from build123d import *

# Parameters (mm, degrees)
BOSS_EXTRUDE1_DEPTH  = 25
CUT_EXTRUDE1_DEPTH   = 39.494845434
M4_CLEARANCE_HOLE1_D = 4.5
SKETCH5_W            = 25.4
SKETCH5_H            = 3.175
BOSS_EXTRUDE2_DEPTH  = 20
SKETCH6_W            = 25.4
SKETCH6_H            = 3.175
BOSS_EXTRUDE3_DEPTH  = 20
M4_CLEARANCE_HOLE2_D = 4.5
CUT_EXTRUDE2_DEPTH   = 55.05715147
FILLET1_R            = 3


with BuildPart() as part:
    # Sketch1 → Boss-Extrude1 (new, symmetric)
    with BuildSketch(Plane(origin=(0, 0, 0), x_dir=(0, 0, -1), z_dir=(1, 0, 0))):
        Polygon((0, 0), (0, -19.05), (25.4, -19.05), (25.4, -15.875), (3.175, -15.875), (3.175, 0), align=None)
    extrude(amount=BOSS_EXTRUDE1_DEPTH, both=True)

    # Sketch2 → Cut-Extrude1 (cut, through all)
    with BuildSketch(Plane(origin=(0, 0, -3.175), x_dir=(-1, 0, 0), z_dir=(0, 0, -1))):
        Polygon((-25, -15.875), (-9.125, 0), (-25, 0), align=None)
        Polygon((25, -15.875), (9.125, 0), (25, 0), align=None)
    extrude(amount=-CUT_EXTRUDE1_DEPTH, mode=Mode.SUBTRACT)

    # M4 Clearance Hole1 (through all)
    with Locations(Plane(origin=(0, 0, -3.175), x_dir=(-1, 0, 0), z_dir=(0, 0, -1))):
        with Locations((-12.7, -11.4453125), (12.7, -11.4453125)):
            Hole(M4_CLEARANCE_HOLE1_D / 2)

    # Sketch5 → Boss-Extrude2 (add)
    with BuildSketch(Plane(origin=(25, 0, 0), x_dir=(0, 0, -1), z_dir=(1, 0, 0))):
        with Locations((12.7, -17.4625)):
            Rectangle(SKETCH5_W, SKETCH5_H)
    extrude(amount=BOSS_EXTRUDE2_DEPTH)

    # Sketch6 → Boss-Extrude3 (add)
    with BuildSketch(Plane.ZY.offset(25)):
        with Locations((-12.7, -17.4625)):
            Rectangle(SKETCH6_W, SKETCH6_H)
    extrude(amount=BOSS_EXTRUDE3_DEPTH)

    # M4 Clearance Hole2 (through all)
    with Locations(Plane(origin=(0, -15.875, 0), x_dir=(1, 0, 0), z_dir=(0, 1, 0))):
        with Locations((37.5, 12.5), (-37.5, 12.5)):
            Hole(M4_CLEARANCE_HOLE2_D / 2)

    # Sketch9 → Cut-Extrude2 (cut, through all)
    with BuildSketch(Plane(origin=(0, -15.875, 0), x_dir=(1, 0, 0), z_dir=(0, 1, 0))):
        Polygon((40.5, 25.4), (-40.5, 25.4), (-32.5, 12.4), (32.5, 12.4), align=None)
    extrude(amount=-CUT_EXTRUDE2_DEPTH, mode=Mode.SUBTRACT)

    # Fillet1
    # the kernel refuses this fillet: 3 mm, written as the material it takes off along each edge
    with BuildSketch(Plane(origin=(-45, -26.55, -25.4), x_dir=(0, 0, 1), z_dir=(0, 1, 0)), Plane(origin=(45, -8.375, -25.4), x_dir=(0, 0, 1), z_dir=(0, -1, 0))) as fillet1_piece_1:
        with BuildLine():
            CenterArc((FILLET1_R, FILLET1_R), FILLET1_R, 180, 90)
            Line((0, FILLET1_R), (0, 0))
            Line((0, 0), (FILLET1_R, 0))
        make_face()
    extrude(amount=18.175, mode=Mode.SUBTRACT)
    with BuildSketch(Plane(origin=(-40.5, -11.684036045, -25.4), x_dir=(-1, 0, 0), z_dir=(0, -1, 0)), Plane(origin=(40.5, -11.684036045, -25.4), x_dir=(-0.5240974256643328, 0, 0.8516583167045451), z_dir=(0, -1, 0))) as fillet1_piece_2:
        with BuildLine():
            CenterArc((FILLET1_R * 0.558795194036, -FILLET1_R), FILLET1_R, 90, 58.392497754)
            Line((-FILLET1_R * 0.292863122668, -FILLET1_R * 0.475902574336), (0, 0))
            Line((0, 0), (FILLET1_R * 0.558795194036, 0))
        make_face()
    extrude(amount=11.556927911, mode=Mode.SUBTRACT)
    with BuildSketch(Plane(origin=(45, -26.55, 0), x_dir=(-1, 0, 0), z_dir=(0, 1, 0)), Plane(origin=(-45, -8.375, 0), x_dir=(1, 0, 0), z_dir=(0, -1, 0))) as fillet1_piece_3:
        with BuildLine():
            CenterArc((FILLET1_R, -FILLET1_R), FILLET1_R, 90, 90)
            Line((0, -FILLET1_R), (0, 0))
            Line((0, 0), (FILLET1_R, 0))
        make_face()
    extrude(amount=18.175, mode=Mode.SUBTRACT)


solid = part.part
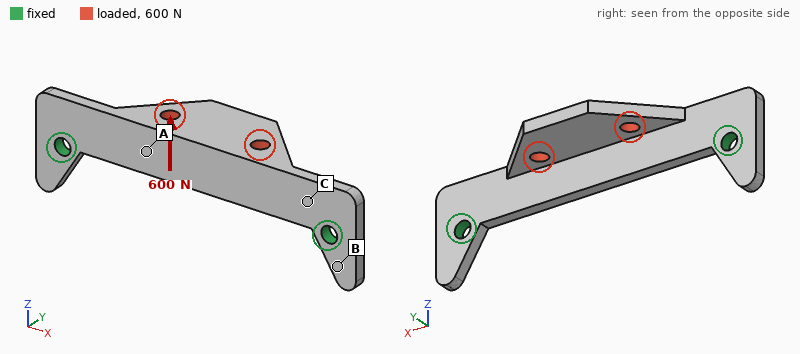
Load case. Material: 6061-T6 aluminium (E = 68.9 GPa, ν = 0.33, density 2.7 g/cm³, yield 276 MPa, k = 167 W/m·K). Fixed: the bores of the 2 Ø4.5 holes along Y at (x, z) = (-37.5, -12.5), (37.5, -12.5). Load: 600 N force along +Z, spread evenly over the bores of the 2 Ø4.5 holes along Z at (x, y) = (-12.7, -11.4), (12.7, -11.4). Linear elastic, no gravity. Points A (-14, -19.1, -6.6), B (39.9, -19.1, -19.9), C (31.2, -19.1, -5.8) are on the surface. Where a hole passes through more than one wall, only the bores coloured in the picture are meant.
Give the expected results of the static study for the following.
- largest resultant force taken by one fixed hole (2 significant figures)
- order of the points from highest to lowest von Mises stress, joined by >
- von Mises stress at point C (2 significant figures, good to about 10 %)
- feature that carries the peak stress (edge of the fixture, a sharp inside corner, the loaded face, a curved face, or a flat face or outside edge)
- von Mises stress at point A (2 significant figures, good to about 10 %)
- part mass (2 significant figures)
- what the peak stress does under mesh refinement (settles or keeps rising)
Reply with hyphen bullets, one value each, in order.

- 460 N
- C > A > B
- 60 MPa
- edge of the fixture
- 27 MPa
- 15 g
- keeps rising
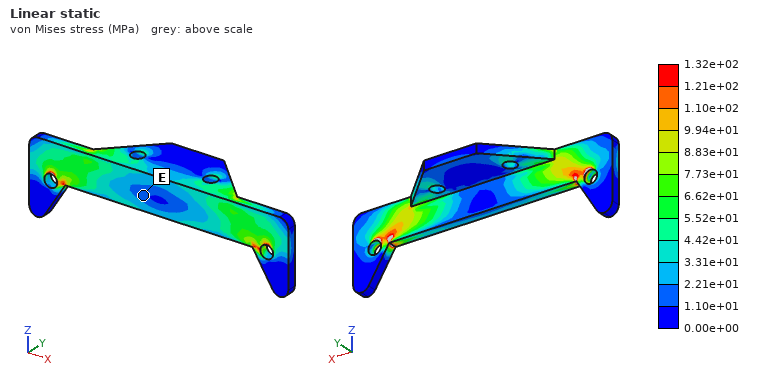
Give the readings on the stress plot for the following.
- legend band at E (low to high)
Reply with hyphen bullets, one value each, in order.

- 1.10e+01 to 2.21e+01 MPa
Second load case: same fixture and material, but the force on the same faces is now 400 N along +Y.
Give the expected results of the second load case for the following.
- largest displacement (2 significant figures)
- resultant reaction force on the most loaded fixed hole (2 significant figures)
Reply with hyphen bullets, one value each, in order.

- 0.16 mm
- 210 N
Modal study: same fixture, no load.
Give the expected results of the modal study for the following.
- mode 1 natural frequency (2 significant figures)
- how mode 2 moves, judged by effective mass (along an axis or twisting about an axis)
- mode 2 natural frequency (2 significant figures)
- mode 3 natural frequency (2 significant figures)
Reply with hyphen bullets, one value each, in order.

- 3000 Hz
- along Y
- 4200 Hz
- 7900 Hz
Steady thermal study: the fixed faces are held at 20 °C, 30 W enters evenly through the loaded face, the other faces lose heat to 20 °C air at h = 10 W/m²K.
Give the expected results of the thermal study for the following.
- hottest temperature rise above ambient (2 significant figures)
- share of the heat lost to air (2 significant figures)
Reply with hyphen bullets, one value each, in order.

- 63 K
- 5.0 %
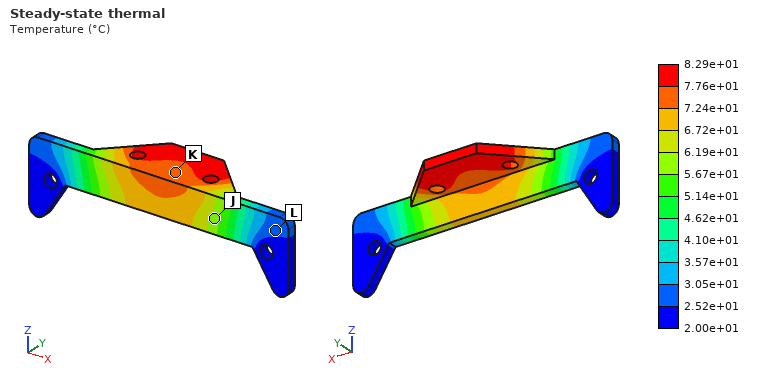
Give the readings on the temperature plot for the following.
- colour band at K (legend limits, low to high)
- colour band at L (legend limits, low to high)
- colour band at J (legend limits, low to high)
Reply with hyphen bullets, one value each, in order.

- 7.24e+01 to 7.76e+01 °C
- 2.52e+01 to 3.05e+01 °C
- 5.67e+01 to 6.19e+01 °C
